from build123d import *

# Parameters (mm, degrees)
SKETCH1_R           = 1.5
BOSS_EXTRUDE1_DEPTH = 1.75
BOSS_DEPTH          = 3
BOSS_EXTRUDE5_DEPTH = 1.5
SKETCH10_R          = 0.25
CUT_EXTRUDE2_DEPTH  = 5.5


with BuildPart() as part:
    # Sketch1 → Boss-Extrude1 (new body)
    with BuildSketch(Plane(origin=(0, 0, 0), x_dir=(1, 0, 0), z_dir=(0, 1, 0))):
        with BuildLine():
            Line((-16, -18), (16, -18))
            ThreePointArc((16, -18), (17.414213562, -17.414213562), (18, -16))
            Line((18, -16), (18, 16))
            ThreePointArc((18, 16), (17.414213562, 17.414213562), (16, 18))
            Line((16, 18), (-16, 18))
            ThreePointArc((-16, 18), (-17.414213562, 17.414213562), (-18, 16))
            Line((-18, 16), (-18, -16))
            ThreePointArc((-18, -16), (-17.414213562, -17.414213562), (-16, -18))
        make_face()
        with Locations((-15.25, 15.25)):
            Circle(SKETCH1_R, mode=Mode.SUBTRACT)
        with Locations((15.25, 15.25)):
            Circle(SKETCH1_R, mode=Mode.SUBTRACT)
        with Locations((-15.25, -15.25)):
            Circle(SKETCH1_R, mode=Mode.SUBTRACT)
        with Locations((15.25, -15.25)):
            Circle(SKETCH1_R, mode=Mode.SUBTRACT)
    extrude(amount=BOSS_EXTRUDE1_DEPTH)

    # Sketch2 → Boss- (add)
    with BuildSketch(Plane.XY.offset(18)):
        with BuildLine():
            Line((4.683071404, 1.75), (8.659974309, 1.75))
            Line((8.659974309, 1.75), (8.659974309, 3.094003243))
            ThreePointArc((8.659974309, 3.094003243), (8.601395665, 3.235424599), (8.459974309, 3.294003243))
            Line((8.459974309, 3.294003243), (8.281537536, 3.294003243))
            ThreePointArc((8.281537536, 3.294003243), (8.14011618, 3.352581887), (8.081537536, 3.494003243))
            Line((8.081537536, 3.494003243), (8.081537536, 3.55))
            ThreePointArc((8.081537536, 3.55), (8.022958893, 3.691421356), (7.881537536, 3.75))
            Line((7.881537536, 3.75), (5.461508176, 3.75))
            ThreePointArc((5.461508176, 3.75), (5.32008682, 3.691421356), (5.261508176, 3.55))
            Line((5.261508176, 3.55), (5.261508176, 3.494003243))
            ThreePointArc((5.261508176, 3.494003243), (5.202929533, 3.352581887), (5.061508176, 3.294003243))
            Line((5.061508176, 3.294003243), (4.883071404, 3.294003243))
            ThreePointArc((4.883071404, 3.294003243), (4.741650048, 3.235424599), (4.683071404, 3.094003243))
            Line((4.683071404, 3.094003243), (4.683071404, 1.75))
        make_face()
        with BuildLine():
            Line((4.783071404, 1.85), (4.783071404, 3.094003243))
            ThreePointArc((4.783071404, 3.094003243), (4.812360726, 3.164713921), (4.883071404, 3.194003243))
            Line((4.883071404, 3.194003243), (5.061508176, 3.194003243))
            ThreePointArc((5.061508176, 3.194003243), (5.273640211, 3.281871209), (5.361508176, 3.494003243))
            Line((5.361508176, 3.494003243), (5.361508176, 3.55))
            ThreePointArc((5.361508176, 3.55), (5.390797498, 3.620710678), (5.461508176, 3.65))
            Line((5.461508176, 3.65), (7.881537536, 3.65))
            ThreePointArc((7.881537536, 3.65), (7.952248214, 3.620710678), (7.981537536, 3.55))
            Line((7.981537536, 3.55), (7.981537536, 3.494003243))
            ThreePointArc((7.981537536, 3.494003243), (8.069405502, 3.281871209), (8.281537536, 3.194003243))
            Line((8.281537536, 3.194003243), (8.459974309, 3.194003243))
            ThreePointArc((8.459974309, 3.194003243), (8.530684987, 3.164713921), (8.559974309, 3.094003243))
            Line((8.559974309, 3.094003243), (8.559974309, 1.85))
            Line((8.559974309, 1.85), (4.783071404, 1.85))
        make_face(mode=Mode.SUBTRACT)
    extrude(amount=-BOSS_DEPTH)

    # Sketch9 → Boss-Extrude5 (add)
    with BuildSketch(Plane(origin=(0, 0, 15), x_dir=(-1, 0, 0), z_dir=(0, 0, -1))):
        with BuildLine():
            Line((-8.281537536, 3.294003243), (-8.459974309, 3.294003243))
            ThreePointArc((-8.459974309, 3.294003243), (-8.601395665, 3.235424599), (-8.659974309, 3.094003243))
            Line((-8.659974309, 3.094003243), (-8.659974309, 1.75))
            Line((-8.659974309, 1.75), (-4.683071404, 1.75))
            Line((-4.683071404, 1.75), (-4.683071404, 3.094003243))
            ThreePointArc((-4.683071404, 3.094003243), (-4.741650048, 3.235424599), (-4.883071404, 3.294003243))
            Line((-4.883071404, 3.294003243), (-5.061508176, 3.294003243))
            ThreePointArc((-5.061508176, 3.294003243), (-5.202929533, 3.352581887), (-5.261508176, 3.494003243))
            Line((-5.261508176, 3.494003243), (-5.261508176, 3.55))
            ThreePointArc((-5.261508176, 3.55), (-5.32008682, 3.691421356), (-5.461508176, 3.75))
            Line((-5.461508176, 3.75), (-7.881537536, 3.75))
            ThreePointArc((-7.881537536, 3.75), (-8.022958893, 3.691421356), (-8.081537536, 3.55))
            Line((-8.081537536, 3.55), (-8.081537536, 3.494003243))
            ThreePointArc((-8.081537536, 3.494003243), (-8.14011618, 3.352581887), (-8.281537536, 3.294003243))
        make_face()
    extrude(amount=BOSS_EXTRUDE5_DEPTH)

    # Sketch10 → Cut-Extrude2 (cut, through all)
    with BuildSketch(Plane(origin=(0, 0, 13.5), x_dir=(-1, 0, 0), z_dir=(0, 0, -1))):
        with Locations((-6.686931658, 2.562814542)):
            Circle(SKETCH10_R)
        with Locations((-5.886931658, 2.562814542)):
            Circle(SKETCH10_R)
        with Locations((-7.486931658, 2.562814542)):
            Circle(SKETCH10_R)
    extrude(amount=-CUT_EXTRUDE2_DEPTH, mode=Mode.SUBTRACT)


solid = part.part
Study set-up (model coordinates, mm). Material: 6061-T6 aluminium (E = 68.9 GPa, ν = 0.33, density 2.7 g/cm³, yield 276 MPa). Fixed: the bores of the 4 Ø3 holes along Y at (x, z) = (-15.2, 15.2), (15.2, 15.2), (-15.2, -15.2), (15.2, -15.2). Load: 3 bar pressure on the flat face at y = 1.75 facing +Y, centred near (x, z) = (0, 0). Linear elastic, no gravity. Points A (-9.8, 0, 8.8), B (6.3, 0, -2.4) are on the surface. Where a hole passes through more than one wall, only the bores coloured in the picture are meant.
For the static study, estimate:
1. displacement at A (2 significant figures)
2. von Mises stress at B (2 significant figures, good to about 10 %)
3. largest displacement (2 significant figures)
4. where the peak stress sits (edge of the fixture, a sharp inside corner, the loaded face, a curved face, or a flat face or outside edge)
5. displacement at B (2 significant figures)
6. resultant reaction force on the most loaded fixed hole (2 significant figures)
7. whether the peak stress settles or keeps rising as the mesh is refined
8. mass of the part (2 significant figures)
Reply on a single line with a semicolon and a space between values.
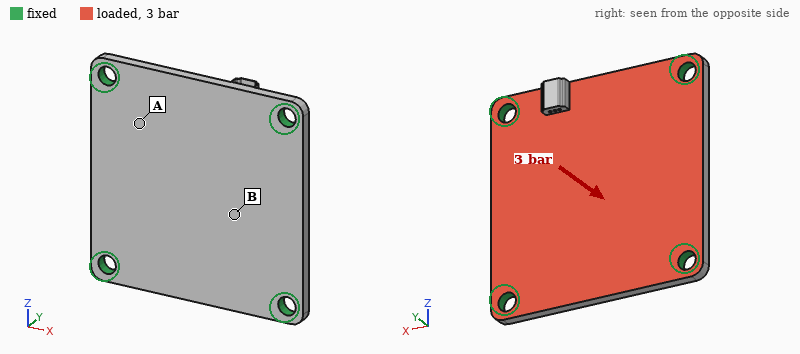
23 µm; 24 MPa; 49 µm; edge of the fixture; 42 µm; 95 N; keeps rising; 6.0 g
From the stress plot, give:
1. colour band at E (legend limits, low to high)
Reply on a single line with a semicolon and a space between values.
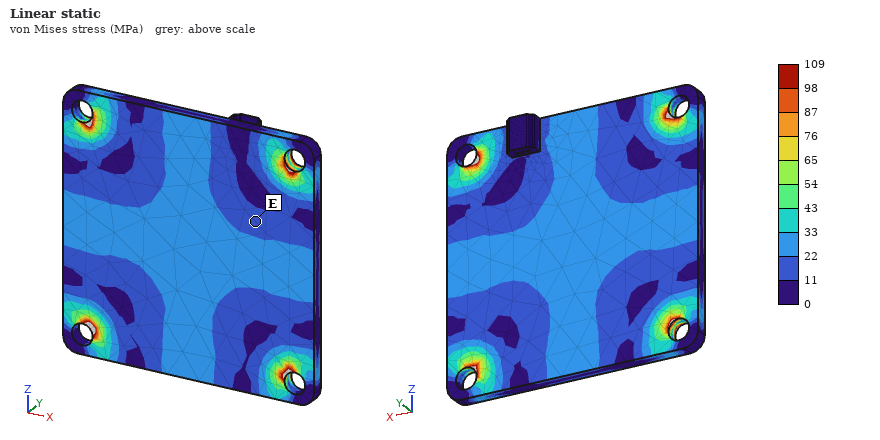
11 to 22 MPa
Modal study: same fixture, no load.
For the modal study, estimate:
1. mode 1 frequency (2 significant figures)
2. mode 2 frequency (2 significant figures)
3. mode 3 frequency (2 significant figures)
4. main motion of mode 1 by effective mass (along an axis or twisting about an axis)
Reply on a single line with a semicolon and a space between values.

7000 Hz; 12 kHz; 12 kHz; along Y
